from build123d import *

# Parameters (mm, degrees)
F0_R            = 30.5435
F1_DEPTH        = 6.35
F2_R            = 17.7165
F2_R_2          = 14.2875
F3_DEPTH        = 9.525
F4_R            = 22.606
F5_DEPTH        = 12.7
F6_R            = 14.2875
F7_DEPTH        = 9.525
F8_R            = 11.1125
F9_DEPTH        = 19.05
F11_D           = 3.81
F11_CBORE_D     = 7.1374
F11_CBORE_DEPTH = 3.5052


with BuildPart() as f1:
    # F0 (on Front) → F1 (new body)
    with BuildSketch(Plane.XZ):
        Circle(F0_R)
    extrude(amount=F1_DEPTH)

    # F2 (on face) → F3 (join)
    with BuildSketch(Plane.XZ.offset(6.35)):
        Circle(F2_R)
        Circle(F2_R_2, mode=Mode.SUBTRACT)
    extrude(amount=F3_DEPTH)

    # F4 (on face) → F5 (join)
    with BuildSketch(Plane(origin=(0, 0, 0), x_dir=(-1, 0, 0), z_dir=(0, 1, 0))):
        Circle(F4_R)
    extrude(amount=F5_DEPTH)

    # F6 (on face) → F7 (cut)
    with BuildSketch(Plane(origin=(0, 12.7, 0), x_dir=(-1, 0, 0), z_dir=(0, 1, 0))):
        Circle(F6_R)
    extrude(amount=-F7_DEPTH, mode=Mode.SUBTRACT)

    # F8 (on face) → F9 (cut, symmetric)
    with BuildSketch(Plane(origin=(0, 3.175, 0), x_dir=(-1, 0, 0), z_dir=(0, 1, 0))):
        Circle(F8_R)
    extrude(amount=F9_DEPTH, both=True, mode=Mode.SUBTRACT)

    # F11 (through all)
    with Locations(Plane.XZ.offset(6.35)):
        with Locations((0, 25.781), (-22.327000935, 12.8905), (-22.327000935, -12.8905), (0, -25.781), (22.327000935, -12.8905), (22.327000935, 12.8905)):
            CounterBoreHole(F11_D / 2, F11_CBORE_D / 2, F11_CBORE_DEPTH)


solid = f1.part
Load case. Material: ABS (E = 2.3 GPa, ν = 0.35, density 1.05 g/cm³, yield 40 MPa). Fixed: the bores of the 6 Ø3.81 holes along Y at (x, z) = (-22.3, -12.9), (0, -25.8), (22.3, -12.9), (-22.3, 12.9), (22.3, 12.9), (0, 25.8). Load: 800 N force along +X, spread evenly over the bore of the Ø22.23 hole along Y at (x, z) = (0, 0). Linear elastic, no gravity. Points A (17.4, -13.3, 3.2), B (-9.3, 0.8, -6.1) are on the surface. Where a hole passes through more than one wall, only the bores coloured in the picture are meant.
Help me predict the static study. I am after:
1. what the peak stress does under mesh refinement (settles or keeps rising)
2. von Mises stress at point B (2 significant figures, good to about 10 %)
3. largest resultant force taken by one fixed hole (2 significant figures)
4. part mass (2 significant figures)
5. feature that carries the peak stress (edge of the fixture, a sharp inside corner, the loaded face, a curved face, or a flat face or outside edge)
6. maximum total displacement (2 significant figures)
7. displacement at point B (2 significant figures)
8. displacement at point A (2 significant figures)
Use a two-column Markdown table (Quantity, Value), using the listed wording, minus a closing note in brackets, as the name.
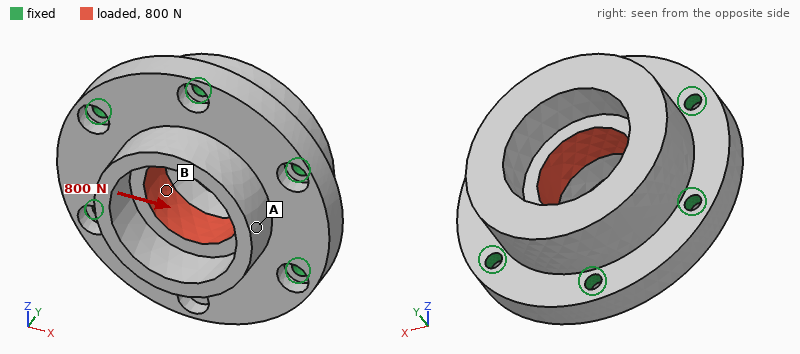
| Quantity | Value |
|---|---|
| what the peak stress does under mesh refinement | keeps rising |
| von Mises stress at point B | 1.4 MPa |
| largest resultant force taken by one fixed hole | 160 N |
| part mass | 33 g |
| feature that carries the peak stress | edge of the fixture |
| maximum total displacement | 17 µm |
| displacement at point B | 16 µm |
| displacement at point A | 12 µm |
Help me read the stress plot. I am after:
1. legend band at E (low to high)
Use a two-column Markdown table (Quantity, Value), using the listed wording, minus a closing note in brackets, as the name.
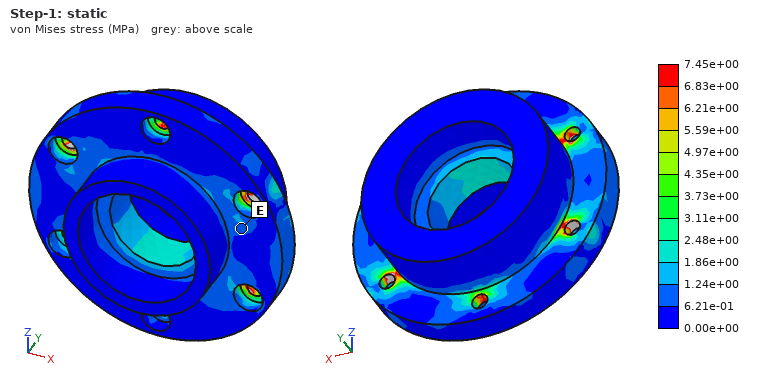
| Quantity | Value |
|---|---|
| legend band at E | 6.21e-01 to 1.24e+00 MPa |
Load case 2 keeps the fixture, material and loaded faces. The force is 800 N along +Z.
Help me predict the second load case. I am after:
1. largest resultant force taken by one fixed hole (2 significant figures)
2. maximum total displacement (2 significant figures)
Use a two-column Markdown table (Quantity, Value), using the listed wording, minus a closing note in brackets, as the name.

| Quantity | Value |
|---|---|
| largest resultant force taken by one fixed hole | 170 N |
| maximum total displacement | 17 µm |
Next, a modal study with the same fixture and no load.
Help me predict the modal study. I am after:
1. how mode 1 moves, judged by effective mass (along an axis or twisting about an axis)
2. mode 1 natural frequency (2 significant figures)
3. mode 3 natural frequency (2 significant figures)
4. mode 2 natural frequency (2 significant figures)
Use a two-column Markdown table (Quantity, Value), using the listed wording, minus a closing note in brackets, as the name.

| Quantity | Value |
|---|---|
| how mode 1 moves, judged by effective mass | along Y |
| mode 1 natural frequency | 5200 Hz |
| mode 3 natural frequency | 6200 Hz |
| mode 2 natural frequency | 6200 Hz |
